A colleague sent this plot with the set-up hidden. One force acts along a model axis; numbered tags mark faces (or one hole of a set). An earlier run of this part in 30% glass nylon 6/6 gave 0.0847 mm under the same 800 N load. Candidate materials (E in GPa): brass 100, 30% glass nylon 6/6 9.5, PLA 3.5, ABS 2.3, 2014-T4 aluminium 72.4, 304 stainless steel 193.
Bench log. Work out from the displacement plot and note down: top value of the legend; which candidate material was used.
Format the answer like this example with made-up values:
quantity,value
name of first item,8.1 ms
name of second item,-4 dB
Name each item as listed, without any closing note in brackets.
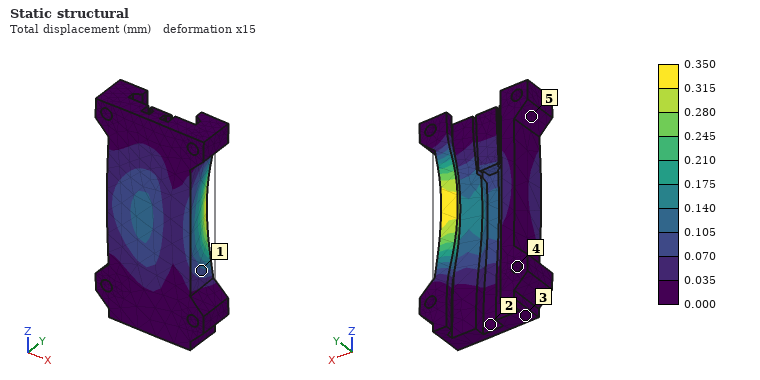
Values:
quantity,value
top value of the legend,0.350 mm
which candidate material was used,ABS
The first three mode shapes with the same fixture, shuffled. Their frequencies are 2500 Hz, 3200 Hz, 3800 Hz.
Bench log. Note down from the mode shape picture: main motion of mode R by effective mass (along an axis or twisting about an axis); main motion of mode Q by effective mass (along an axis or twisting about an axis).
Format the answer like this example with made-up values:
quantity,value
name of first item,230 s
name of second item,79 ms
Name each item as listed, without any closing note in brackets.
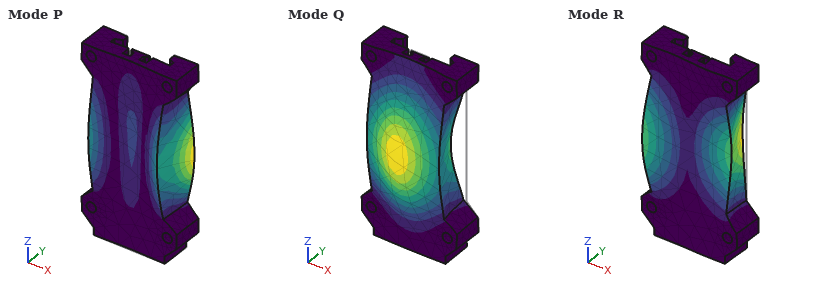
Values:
quantity,value
main motion of mode R by effective mass,along X
main motion of mode Q by effective mass,along Y
